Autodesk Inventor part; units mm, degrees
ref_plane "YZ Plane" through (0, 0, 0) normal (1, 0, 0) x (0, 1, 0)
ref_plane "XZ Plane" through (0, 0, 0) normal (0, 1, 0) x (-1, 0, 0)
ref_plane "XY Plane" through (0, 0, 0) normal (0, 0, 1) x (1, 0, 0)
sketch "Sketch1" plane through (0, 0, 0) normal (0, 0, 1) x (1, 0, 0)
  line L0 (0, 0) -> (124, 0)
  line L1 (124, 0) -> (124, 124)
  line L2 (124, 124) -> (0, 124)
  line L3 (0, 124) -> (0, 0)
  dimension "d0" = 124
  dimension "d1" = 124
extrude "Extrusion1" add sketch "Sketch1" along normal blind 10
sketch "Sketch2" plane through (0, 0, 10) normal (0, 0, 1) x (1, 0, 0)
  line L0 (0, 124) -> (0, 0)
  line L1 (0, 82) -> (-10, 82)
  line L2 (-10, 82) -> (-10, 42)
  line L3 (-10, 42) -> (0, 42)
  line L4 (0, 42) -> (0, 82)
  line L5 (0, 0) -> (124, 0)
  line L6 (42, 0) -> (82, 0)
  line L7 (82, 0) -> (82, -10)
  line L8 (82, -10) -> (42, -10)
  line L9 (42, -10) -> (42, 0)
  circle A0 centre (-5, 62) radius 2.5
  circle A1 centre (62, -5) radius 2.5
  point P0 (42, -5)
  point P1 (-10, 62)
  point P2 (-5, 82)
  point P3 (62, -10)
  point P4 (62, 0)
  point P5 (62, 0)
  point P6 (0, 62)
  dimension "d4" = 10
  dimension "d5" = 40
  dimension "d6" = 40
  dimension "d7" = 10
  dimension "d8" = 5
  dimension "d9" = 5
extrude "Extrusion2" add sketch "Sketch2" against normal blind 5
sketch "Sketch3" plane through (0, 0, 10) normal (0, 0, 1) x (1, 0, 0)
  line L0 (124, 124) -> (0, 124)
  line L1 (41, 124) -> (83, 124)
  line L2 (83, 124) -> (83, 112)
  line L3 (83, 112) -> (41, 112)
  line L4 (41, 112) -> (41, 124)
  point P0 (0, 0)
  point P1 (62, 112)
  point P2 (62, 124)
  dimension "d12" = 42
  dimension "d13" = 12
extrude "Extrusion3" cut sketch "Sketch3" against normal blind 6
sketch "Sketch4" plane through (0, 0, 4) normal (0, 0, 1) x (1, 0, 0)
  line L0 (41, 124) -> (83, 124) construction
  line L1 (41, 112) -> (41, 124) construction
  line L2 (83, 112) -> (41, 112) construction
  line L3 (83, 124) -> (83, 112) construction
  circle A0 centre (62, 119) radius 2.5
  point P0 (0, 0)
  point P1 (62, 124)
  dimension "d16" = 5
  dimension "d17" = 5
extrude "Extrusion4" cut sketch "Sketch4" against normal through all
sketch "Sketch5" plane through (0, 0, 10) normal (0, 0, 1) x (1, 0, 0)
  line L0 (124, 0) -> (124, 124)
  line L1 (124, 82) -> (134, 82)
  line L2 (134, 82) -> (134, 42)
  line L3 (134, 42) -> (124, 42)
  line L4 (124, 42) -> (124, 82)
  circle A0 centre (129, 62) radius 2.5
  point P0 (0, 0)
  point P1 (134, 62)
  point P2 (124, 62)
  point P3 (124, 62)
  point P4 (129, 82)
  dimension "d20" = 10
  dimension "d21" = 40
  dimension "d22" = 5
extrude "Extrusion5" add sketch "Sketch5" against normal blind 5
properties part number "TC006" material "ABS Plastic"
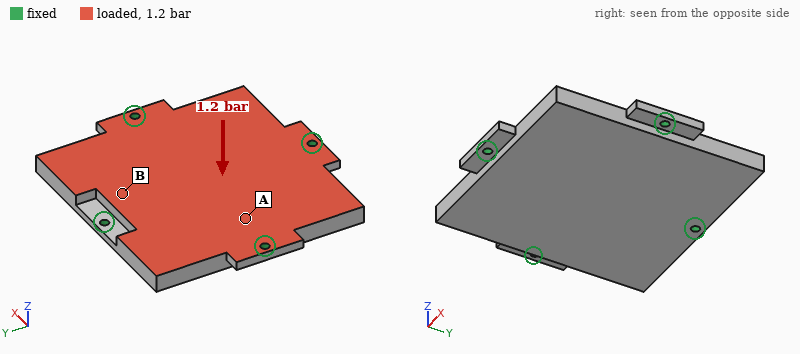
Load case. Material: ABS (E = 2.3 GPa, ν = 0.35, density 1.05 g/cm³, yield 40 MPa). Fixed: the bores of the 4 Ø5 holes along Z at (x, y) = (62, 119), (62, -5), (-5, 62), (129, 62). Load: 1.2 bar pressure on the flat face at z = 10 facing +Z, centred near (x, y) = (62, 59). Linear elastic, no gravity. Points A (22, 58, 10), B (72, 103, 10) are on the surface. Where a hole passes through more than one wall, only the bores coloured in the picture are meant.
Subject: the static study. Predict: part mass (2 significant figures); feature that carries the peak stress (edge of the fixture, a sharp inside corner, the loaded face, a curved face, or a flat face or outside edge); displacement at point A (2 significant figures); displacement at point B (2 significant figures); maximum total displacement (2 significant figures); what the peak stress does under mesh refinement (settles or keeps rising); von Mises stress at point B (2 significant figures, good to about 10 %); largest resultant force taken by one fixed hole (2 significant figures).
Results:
160 g
edge of the fixture
0.36 mm
0.32 mm
0.53 mm
keeps rising
6.3 MPa
660 N
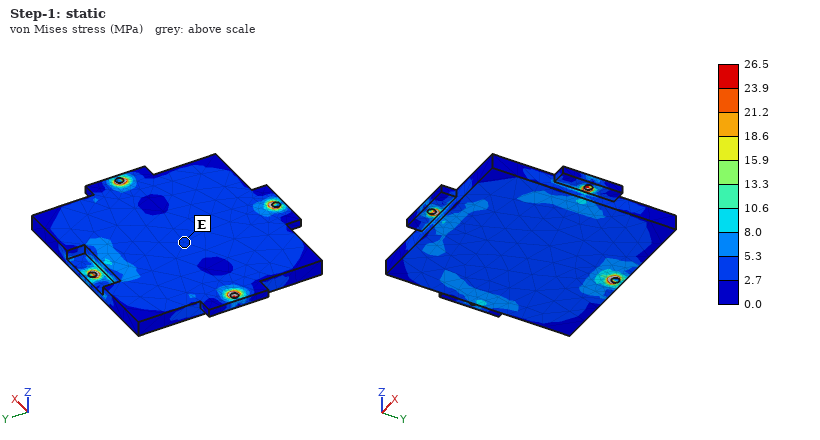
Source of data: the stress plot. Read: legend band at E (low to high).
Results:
2.7 to 5.3 MPa
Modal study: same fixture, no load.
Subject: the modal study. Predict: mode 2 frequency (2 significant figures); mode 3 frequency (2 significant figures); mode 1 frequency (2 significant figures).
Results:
840 Hz
850 Hz
730 Hz
